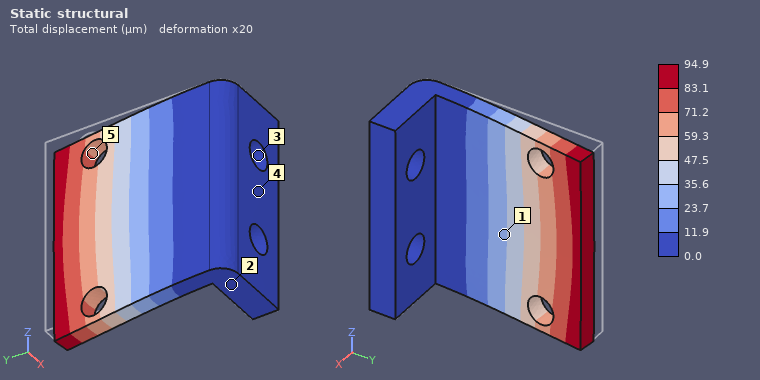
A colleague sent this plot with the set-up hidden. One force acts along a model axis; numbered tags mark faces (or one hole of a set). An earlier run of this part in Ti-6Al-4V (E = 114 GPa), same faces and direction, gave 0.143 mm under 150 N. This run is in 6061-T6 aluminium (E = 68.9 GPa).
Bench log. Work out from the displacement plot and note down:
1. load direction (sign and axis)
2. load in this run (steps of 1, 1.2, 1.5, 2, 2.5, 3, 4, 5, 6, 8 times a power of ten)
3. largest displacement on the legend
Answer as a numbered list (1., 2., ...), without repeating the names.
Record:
1. +X
2. 60 N
3. 94.9 µm
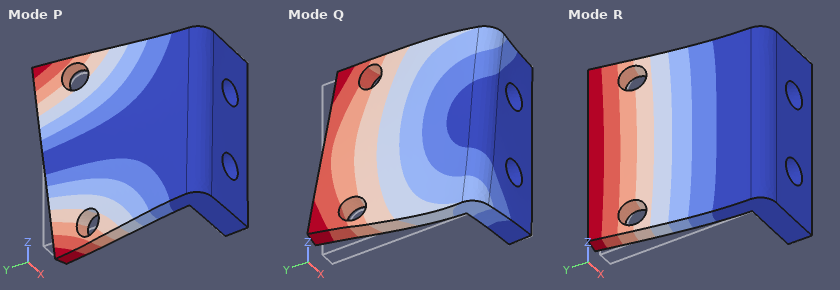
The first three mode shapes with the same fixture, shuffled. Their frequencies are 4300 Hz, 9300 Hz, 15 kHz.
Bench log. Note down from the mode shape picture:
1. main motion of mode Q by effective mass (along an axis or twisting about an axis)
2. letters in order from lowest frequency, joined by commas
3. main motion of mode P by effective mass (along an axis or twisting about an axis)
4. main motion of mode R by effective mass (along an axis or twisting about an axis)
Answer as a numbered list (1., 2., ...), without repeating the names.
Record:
1. along Z
2. R, P, Q
3. twisting about Y
4. along X
